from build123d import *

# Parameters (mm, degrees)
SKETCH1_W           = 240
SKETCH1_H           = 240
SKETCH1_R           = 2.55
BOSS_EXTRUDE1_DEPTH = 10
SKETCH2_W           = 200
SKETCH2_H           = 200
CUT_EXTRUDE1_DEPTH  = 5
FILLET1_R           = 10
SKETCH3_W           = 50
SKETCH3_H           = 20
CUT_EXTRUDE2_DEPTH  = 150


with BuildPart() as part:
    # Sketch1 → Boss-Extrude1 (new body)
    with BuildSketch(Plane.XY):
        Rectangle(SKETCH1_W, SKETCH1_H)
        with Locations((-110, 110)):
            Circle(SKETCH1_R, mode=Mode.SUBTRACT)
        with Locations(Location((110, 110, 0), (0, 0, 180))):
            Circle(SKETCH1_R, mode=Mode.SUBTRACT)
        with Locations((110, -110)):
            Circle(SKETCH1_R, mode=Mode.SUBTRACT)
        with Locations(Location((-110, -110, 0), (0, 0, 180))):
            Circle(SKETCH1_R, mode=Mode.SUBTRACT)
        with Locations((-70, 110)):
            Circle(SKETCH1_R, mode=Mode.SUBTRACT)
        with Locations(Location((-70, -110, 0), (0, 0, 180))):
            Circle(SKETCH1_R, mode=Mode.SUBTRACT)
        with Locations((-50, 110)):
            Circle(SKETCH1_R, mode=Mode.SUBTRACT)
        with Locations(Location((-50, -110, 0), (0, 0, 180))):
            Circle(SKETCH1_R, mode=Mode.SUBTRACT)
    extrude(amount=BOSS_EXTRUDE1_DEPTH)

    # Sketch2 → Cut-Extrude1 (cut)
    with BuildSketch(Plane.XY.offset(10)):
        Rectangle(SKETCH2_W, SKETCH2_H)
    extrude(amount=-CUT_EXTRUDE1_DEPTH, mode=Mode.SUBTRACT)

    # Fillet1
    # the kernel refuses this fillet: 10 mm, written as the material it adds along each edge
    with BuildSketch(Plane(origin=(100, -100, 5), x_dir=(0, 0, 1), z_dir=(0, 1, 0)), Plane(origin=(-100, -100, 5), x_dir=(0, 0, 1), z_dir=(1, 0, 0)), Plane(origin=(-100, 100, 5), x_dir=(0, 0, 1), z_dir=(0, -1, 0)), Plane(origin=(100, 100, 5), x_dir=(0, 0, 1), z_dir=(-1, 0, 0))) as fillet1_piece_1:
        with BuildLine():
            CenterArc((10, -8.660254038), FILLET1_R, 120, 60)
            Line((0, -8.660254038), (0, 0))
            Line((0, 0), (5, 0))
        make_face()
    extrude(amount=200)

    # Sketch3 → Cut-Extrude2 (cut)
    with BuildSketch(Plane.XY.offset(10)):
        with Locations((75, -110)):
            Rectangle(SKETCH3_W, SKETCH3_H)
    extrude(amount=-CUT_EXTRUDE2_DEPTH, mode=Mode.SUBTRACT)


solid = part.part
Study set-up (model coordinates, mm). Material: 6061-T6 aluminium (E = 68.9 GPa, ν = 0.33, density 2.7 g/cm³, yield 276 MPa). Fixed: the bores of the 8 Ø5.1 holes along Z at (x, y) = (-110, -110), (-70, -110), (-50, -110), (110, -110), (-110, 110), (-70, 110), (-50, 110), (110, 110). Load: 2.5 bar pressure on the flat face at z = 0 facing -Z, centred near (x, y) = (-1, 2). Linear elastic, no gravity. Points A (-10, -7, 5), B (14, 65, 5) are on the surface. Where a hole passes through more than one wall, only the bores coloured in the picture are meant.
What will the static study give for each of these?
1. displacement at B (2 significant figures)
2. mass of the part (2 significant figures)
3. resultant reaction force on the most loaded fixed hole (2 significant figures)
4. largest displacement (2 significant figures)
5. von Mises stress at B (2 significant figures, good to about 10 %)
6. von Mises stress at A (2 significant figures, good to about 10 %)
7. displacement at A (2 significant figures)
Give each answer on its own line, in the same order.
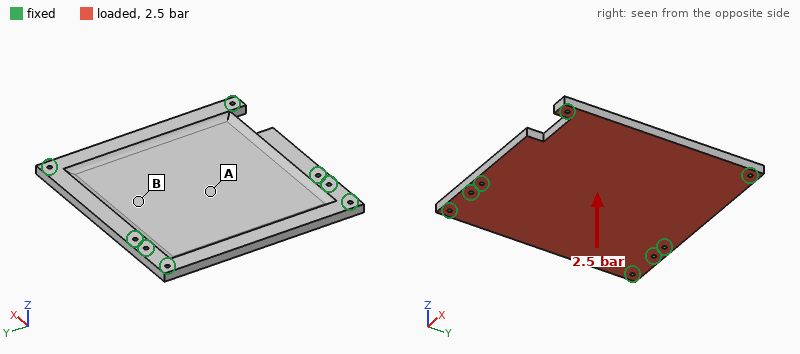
0.83 mm
1.0 kg
5.4 kN
1.5 mm
30 MPa
72 MPa
1.4 mm
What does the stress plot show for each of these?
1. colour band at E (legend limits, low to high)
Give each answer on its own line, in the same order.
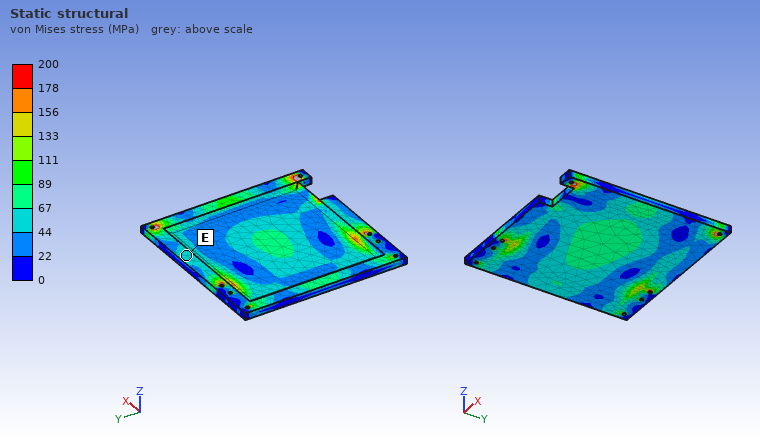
44 to 67 MPa
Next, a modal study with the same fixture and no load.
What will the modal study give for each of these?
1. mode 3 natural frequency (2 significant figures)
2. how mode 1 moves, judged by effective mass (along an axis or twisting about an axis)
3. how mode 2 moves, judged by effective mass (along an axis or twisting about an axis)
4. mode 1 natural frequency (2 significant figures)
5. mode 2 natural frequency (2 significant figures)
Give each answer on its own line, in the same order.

1200 Hz
along Z
twisting about Y
680 Hz
960 Hz
